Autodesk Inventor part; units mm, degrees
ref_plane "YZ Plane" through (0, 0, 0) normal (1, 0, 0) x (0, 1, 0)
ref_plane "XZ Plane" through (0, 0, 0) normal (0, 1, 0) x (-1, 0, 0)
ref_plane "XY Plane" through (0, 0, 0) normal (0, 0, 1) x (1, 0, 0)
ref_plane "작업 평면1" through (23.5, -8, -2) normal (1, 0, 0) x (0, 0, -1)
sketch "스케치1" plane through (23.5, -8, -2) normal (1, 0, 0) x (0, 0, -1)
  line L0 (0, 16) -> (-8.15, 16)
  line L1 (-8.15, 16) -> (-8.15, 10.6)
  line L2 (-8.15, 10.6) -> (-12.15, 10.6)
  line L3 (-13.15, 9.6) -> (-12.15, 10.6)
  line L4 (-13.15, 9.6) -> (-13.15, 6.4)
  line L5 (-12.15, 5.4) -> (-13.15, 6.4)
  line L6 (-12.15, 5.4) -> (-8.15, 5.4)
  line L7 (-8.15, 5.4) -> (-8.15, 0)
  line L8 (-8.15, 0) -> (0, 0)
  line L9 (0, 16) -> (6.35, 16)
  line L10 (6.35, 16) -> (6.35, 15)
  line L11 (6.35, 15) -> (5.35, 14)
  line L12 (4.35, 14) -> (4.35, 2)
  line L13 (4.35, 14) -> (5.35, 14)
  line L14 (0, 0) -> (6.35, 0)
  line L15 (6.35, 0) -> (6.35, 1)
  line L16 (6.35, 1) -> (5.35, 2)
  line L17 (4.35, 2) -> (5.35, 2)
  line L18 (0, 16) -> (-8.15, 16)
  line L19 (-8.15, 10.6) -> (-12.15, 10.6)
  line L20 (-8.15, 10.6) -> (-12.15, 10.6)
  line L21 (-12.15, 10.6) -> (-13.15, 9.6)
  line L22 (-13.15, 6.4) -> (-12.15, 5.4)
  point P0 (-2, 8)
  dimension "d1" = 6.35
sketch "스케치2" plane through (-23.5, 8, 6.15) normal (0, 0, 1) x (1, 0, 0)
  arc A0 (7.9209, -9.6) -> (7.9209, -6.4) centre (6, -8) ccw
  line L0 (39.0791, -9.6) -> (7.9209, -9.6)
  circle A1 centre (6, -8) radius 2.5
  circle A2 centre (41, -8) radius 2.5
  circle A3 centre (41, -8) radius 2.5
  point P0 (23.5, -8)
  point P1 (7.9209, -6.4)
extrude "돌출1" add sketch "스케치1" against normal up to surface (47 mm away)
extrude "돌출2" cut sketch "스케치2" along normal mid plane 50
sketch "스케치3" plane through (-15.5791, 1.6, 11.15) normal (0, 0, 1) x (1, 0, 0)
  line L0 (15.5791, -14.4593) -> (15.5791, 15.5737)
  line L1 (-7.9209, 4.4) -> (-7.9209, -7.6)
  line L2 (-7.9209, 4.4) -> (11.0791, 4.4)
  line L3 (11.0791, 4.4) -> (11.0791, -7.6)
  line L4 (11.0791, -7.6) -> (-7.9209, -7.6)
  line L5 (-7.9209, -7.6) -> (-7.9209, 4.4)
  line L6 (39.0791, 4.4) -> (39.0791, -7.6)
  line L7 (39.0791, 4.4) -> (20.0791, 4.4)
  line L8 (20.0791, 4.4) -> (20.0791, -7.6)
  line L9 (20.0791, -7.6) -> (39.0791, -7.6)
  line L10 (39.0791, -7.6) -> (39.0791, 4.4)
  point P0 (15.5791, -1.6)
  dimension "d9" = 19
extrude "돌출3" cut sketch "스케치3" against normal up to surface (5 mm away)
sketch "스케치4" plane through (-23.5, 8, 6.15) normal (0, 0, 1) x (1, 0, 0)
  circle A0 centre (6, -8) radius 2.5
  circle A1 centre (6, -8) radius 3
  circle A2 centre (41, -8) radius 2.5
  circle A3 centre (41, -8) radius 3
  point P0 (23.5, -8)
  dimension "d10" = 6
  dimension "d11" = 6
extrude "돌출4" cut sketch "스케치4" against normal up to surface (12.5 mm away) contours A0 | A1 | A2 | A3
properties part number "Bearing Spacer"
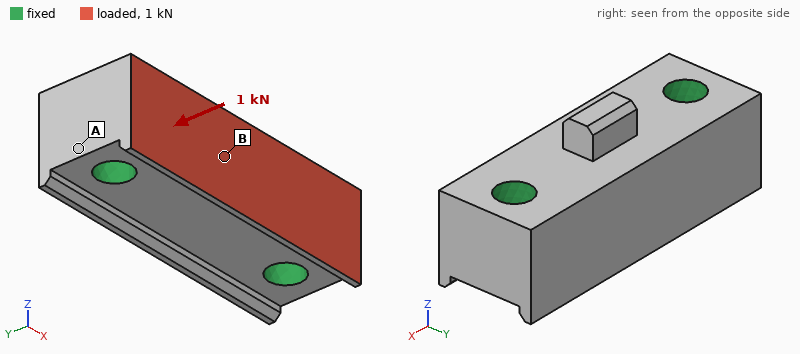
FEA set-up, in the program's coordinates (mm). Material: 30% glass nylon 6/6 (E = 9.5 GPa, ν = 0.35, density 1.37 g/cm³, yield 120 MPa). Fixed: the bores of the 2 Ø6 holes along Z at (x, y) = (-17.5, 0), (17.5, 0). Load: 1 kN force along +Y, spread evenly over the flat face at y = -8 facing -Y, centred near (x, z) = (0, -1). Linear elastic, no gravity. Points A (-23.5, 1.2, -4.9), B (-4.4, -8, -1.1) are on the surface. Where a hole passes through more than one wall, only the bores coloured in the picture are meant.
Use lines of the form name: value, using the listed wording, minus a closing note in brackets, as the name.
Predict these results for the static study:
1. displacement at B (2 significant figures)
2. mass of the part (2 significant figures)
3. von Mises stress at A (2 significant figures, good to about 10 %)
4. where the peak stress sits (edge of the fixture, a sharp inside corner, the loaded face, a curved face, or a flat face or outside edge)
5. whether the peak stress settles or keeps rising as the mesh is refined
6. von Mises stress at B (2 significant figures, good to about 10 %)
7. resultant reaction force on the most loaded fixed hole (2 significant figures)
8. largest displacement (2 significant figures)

displacement at B: 7.3 µm
mass of the part: 13 g
von Mises stress at A: 1.3 MPa
where the peak stress sits: edge of the fixture
whether the peak stress settles or keeps rising as the mesh is refined: keeps rising
von Mises stress at B: 3.2 MPa
resultant reaction force on the most loaded fixed hole: 500 N
largest displacement: 13 µm
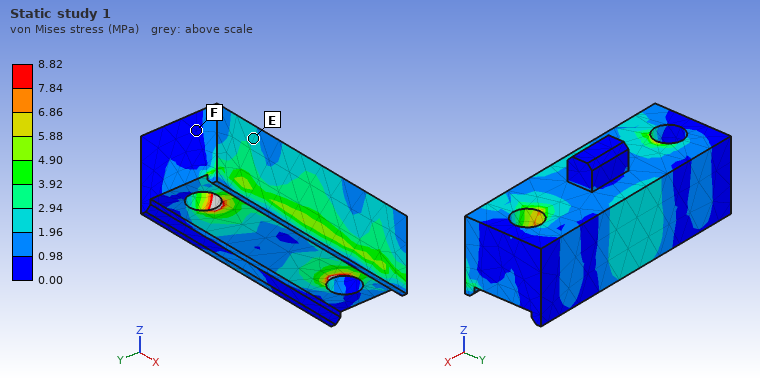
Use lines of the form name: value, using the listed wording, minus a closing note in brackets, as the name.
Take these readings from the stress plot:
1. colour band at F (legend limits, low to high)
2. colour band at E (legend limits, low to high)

colour band at F: 0.00 to 0.98 MPa
colour band at E: 1.96 to 2.94 MPa
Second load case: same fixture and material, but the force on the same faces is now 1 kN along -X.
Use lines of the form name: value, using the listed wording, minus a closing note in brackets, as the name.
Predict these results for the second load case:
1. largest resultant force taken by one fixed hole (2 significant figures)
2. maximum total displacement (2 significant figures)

largest resultant force taken by one fixed hole: 530 N
maximum total displacement: 8.7 µm
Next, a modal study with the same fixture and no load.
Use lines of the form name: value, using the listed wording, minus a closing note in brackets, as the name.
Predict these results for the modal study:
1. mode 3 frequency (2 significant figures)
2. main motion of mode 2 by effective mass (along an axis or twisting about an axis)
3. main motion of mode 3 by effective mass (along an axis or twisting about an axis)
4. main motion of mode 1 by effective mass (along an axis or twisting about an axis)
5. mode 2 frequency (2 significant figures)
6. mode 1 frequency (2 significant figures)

mode 3 frequency: 20 kHz
main motion of mode 2 by effective mass: along Z
main motion of mode 3 by effective mass: twisting about X
main motion of mode 1 by effective mass: along Y
mode 2 frequency: 18 kHz
mode 1 frequency: 17 kHz
